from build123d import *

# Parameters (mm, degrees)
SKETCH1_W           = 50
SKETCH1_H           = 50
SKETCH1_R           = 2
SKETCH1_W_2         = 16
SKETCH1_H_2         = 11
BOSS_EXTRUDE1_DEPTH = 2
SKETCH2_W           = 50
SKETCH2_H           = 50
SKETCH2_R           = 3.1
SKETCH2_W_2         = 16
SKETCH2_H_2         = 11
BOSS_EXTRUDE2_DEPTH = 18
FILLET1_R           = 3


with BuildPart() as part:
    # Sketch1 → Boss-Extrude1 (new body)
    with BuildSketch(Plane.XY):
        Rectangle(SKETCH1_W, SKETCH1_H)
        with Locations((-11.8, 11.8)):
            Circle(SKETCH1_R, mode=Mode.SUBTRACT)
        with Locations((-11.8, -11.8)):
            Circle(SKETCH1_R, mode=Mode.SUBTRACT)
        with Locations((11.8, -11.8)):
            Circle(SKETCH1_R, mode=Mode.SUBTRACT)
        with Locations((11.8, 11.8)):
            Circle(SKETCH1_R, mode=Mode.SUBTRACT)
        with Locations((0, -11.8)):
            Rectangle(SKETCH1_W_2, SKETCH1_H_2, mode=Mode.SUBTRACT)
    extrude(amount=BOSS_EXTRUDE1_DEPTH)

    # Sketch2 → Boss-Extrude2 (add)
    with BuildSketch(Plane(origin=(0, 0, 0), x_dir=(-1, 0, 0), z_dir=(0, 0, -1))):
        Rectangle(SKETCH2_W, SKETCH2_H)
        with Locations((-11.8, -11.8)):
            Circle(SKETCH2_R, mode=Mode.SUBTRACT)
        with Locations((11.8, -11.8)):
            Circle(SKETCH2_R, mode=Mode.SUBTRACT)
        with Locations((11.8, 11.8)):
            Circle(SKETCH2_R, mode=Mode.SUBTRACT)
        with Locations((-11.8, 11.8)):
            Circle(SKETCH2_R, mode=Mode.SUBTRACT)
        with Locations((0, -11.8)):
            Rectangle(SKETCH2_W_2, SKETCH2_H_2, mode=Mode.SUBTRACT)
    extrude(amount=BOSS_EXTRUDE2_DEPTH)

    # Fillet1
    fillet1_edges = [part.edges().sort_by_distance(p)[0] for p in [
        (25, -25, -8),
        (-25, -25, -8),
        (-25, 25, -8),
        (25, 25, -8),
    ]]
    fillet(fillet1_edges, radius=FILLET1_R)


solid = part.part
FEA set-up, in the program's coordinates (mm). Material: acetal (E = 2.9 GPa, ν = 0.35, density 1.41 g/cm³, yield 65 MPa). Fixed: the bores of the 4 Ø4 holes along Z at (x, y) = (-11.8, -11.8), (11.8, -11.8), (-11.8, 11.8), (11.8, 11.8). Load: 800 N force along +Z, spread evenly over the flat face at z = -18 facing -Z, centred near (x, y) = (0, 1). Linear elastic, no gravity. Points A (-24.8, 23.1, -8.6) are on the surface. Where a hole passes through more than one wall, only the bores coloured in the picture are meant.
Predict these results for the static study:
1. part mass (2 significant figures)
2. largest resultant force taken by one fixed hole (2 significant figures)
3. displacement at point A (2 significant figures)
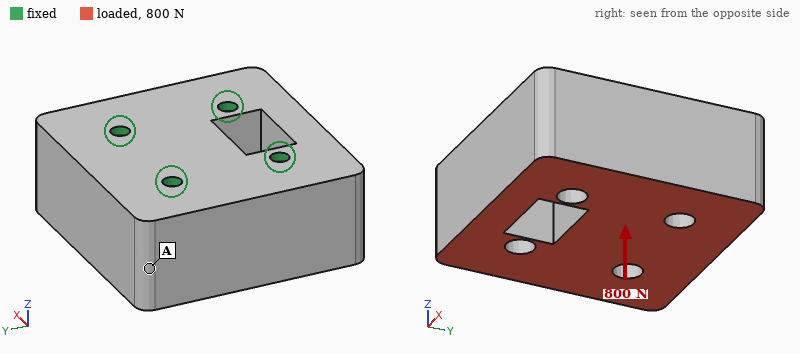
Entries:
62 g
220 N
23 µm
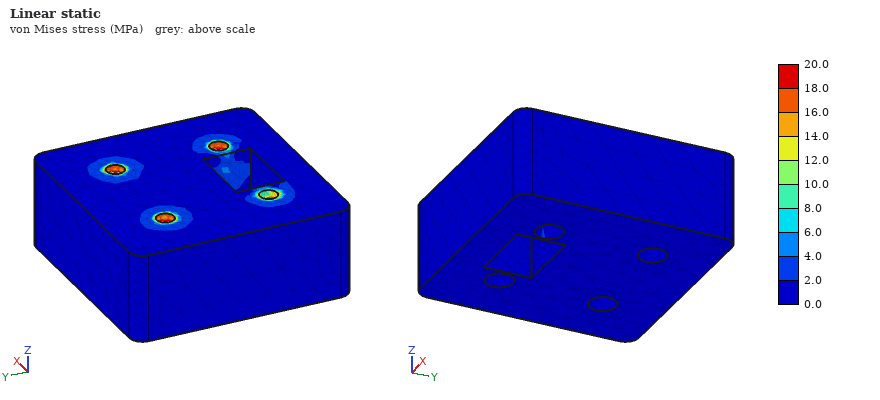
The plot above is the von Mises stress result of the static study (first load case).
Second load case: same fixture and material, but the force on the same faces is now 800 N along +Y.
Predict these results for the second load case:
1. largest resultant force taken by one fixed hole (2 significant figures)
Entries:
370 N
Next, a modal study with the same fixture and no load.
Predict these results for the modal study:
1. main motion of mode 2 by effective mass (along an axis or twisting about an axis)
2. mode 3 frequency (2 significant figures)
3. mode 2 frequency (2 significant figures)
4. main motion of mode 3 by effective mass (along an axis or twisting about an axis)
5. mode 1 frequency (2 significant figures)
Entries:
along Y
3900 Hz
2500 Hz
twisting about Z
2400 Hz
